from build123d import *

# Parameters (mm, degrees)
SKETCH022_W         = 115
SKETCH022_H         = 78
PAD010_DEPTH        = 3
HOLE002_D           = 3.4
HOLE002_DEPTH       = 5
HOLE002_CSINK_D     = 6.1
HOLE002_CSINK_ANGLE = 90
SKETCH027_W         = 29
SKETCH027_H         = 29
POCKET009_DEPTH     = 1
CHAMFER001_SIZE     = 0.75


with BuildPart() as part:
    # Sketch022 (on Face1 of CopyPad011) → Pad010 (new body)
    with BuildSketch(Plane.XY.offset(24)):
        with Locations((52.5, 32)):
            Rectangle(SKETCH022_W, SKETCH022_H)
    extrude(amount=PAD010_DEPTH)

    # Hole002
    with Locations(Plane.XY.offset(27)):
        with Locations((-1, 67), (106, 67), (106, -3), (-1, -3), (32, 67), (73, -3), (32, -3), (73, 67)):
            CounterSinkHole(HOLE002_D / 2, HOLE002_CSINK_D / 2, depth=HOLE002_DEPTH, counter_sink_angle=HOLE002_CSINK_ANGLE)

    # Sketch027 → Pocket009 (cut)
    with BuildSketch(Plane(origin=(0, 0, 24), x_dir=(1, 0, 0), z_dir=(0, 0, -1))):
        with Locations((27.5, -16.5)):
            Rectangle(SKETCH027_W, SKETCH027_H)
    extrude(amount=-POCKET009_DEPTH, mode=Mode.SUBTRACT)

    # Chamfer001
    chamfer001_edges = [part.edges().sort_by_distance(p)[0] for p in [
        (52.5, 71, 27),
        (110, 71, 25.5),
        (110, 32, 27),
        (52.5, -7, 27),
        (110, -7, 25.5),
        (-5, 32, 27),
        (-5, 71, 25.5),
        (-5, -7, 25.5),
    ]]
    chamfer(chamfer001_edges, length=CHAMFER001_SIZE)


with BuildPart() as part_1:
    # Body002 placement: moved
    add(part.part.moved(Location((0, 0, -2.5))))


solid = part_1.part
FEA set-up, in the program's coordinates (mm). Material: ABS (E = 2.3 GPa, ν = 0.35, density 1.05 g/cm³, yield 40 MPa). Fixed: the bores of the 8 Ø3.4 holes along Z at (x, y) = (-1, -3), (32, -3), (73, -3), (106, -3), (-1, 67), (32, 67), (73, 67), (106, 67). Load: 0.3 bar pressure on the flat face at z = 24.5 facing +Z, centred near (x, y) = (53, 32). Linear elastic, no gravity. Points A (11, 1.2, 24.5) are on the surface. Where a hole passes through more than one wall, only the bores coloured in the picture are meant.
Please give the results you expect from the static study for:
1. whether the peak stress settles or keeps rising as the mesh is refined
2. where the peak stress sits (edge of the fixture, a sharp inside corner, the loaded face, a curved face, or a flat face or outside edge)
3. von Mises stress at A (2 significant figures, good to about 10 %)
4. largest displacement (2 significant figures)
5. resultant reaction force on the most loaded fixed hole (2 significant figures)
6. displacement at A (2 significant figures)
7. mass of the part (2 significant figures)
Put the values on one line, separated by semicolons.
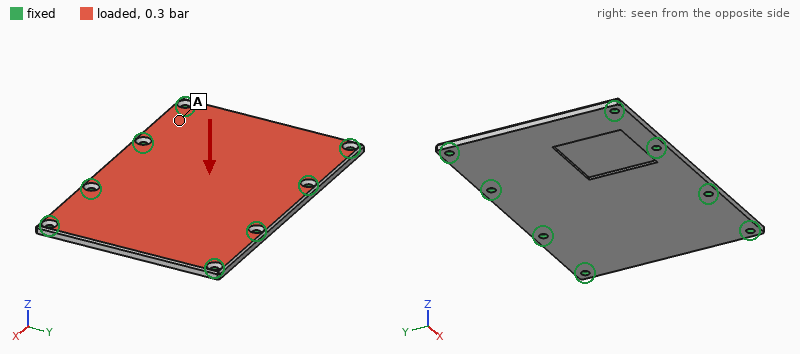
keeps rising; edge of the fixture; 3.2 MPa; 0.71 mm; 64 N; 0.11 mm; 27 g
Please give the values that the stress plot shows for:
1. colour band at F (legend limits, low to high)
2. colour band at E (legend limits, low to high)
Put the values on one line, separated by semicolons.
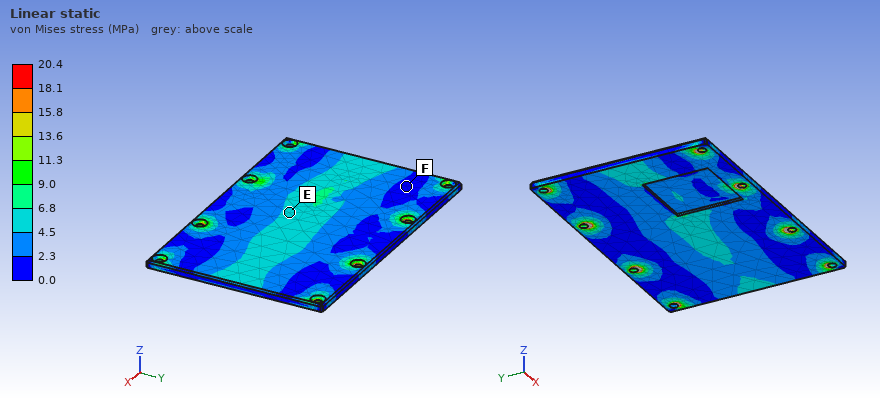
0.0 to 2.3 MPa; 4.5 to 6.8 MPa
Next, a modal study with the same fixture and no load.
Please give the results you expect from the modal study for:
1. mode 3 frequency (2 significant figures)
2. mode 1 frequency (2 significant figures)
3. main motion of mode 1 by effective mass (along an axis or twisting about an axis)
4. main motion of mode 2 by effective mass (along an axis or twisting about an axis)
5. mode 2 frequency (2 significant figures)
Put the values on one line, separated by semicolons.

1100 Hz; 720 Hz; along Z; twisting about Y; 840 Hz
